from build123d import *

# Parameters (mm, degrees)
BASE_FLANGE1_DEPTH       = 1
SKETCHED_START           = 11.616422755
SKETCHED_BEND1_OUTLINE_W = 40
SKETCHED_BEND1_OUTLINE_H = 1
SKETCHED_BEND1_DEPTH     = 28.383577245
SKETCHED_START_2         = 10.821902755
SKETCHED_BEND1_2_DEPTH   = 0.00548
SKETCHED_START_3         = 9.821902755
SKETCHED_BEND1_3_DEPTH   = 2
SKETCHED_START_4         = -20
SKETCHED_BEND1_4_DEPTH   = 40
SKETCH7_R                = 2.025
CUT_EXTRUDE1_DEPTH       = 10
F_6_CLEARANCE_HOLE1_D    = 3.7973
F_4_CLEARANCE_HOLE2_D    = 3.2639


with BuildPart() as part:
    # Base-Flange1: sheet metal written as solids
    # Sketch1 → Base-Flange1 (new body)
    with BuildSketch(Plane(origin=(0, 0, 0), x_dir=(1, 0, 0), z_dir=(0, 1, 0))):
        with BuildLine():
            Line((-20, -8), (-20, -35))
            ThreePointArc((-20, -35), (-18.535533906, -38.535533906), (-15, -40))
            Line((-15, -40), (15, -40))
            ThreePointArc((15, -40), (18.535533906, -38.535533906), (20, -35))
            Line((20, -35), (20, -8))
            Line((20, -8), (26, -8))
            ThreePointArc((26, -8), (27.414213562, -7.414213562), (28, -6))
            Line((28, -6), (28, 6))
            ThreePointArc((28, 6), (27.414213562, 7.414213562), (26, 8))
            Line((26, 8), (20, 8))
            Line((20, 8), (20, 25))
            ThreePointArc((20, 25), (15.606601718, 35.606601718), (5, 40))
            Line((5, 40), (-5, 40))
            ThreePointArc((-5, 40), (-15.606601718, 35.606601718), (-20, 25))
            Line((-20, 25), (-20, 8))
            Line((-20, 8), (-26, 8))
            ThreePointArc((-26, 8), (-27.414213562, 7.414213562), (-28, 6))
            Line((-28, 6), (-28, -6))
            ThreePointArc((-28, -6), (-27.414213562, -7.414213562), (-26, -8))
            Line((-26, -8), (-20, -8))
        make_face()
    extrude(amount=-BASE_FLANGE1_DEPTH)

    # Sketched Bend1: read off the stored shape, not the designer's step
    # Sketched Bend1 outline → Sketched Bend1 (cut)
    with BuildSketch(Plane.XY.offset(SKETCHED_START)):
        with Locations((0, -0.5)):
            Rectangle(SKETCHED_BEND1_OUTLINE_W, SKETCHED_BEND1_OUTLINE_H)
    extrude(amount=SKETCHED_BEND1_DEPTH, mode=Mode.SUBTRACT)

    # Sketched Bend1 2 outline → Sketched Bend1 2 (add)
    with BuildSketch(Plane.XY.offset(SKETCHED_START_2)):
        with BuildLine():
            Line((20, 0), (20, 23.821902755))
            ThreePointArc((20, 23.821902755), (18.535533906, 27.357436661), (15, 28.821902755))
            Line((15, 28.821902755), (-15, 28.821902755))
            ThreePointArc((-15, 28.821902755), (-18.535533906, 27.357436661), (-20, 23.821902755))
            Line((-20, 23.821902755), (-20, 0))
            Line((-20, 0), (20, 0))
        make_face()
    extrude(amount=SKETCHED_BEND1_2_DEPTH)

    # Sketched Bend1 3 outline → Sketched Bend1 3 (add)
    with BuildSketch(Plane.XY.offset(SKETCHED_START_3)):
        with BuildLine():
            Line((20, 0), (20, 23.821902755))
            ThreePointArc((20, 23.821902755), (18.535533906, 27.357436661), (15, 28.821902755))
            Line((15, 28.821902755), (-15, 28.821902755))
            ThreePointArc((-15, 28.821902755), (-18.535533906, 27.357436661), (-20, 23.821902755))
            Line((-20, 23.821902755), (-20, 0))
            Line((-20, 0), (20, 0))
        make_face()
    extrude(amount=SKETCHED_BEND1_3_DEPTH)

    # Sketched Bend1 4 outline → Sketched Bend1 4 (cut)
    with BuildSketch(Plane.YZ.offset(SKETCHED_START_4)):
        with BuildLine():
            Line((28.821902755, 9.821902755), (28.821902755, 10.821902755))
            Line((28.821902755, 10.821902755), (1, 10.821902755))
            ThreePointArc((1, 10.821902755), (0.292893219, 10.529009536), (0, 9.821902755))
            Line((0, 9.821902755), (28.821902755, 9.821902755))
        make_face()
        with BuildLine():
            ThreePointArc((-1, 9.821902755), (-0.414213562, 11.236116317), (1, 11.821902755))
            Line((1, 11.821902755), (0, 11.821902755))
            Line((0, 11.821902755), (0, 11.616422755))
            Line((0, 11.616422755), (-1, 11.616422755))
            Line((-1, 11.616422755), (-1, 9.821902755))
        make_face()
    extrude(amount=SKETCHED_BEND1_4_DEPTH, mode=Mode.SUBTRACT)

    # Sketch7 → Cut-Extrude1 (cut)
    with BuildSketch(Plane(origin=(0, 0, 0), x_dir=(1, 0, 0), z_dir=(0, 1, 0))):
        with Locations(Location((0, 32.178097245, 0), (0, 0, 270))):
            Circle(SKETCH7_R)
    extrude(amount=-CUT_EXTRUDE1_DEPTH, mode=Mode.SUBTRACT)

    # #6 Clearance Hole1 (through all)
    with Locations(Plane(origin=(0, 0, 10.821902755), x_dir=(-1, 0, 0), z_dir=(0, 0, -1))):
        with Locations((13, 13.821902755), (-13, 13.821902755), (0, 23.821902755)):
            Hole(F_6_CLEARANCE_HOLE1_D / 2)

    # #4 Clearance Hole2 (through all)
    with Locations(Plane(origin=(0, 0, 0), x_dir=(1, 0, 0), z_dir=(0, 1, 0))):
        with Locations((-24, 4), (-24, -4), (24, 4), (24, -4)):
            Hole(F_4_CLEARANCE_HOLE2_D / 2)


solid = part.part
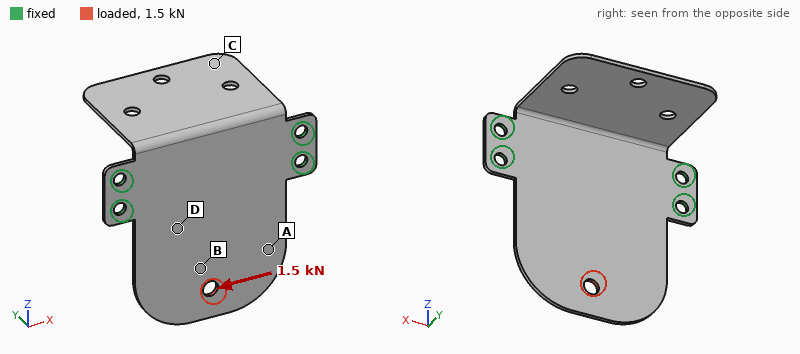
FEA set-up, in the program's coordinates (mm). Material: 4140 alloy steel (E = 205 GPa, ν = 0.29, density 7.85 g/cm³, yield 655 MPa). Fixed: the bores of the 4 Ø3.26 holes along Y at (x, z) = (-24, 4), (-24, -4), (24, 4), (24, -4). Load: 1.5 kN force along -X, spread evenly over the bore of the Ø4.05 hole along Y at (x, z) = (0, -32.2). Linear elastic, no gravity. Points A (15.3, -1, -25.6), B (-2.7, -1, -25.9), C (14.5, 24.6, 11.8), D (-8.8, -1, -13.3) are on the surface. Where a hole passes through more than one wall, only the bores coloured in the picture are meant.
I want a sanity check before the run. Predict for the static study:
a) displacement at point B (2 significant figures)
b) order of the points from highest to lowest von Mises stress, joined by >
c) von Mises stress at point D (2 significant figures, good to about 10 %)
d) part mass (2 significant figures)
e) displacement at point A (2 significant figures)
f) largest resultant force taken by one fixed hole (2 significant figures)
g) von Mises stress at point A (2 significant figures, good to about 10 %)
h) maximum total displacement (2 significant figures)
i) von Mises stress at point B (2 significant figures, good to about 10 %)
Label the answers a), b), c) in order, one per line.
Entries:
a) 24 µm
b) B > D > A > C
c) 78 MPa
d) 26 g
e) 25 µm
f) 760 N
g) 48 MPa
h) 38 µm
i) 100 MPa
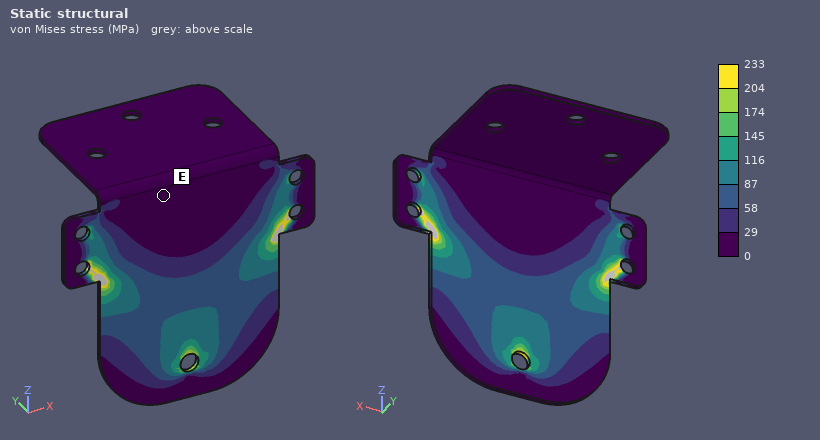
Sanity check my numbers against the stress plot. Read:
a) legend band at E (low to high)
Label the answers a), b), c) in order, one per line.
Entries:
a) 0 to 29 MPa
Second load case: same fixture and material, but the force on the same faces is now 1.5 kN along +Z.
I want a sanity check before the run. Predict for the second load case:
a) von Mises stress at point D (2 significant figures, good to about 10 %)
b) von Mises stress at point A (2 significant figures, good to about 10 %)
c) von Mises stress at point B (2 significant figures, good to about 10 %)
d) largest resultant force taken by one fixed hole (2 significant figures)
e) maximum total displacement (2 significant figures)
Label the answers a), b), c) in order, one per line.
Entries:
a) 43 MPa
b) 23 MPa
c) 82 MPa
d) 430 N
e) 16 µm
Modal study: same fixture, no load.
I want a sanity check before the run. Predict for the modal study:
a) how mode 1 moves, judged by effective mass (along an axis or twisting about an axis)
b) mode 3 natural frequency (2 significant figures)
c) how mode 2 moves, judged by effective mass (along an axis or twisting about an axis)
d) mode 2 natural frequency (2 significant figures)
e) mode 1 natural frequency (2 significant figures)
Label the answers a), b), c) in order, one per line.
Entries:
a) along Y
b) 1600 Hz
c) along Z
d) 680 Hz
e) 550 Hz
